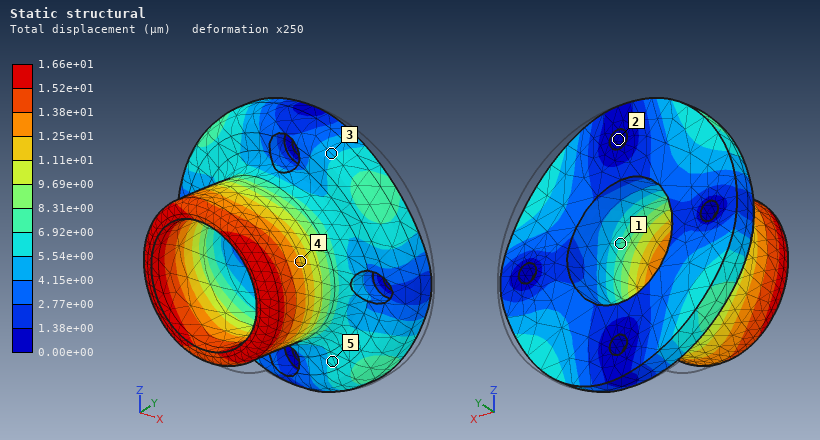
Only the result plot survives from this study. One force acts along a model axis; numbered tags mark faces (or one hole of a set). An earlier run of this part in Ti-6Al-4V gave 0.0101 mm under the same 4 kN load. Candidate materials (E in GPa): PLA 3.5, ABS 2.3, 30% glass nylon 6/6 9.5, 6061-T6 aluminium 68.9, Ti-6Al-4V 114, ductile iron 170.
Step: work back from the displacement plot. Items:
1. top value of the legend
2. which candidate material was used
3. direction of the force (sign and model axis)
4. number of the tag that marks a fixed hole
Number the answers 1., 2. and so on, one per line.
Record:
1. 1.66e+01 µm
2. 6061-T6 aluminium
3. -X
4. 2
